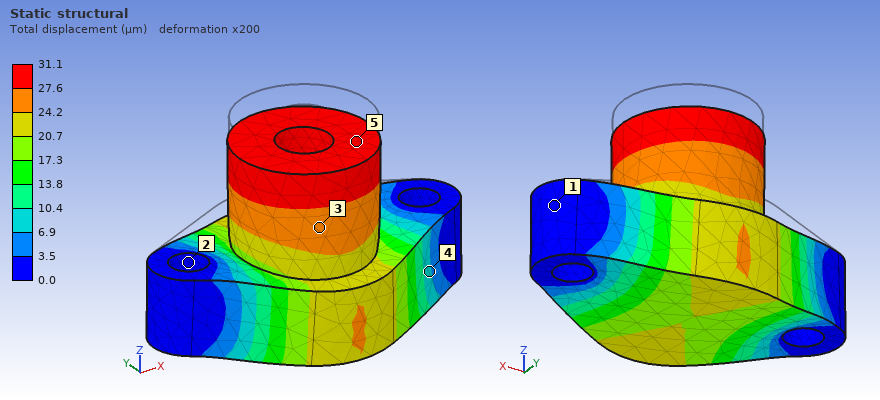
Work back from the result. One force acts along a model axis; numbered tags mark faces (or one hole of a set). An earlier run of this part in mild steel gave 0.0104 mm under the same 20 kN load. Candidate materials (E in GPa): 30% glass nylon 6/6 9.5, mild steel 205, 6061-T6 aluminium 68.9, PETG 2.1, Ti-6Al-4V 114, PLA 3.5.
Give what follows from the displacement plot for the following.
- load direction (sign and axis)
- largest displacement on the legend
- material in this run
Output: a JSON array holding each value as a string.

["-Z", "31.1 µm", "6061-T6 aluminium"]
